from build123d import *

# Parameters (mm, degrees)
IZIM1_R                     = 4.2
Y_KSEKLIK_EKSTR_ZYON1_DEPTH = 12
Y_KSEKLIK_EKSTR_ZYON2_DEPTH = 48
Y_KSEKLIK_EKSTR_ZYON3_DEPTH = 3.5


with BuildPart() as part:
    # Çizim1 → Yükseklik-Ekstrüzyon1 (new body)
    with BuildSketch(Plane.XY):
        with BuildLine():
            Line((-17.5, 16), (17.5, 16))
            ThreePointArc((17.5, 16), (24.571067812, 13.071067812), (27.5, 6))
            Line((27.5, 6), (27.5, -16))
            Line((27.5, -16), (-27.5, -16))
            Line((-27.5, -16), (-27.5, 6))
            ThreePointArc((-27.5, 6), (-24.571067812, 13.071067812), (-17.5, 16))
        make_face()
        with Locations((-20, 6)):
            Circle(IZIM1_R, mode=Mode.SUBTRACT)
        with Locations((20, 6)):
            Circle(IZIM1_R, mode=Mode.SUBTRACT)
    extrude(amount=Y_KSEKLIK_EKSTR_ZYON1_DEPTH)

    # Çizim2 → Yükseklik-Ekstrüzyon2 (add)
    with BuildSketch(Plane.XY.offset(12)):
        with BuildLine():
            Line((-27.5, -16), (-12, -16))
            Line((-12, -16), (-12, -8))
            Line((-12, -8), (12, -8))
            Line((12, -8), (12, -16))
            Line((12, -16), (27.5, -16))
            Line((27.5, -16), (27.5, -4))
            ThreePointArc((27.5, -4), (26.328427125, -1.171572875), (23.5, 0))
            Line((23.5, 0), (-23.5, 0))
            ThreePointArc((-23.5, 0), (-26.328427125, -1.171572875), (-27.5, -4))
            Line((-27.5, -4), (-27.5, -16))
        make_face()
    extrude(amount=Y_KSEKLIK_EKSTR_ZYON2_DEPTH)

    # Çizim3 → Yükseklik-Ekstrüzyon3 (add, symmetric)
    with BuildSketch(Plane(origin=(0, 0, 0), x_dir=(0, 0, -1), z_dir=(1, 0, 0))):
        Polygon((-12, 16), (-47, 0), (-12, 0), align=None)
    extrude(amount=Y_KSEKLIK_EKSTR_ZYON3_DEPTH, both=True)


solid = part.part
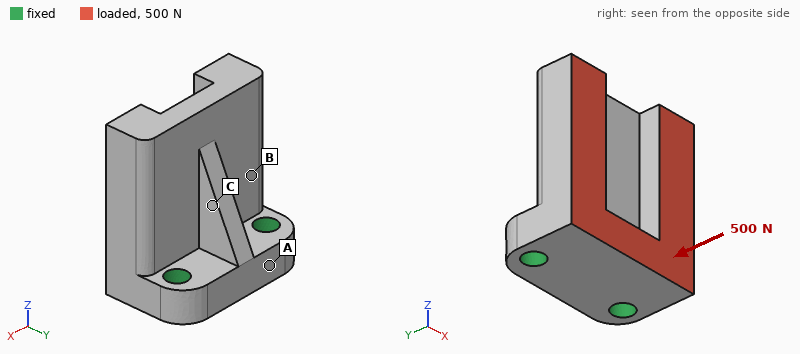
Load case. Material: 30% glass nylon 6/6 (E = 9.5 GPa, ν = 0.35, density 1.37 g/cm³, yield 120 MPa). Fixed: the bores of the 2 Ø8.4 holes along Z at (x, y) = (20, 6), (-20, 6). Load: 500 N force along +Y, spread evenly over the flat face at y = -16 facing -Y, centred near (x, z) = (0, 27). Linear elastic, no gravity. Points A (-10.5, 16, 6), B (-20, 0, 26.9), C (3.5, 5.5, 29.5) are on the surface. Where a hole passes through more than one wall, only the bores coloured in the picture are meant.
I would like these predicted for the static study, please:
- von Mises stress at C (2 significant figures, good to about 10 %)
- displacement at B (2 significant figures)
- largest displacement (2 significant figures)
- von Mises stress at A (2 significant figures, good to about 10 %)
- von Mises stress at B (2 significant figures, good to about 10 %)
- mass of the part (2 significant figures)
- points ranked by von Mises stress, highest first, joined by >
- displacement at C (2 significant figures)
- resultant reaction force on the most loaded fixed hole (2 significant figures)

3.1 MPa
0.033 mm
0.11 mm
4.6 MPa
1.2 MPa
74 g
A > C > B
0.035 mm
250 N
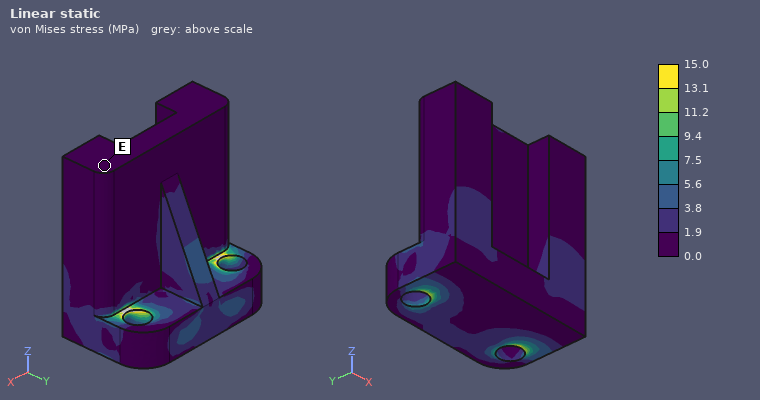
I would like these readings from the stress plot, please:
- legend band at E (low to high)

0.0 to 1.9 MPa
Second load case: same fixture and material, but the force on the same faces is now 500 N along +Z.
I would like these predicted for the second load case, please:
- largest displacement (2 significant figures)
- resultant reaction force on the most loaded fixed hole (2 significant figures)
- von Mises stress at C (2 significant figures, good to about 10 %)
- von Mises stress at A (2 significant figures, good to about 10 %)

79 µm
250 N
1.6 MPa
3.4 MPa
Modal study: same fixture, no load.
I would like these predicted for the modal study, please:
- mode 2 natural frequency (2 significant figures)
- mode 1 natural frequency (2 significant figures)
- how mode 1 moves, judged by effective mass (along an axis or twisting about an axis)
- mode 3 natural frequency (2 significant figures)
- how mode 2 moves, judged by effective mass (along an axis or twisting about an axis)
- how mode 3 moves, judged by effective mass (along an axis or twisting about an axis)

3100 Hz
1700 Hz
along Y
3500 Hz
twisting about Z
along X
